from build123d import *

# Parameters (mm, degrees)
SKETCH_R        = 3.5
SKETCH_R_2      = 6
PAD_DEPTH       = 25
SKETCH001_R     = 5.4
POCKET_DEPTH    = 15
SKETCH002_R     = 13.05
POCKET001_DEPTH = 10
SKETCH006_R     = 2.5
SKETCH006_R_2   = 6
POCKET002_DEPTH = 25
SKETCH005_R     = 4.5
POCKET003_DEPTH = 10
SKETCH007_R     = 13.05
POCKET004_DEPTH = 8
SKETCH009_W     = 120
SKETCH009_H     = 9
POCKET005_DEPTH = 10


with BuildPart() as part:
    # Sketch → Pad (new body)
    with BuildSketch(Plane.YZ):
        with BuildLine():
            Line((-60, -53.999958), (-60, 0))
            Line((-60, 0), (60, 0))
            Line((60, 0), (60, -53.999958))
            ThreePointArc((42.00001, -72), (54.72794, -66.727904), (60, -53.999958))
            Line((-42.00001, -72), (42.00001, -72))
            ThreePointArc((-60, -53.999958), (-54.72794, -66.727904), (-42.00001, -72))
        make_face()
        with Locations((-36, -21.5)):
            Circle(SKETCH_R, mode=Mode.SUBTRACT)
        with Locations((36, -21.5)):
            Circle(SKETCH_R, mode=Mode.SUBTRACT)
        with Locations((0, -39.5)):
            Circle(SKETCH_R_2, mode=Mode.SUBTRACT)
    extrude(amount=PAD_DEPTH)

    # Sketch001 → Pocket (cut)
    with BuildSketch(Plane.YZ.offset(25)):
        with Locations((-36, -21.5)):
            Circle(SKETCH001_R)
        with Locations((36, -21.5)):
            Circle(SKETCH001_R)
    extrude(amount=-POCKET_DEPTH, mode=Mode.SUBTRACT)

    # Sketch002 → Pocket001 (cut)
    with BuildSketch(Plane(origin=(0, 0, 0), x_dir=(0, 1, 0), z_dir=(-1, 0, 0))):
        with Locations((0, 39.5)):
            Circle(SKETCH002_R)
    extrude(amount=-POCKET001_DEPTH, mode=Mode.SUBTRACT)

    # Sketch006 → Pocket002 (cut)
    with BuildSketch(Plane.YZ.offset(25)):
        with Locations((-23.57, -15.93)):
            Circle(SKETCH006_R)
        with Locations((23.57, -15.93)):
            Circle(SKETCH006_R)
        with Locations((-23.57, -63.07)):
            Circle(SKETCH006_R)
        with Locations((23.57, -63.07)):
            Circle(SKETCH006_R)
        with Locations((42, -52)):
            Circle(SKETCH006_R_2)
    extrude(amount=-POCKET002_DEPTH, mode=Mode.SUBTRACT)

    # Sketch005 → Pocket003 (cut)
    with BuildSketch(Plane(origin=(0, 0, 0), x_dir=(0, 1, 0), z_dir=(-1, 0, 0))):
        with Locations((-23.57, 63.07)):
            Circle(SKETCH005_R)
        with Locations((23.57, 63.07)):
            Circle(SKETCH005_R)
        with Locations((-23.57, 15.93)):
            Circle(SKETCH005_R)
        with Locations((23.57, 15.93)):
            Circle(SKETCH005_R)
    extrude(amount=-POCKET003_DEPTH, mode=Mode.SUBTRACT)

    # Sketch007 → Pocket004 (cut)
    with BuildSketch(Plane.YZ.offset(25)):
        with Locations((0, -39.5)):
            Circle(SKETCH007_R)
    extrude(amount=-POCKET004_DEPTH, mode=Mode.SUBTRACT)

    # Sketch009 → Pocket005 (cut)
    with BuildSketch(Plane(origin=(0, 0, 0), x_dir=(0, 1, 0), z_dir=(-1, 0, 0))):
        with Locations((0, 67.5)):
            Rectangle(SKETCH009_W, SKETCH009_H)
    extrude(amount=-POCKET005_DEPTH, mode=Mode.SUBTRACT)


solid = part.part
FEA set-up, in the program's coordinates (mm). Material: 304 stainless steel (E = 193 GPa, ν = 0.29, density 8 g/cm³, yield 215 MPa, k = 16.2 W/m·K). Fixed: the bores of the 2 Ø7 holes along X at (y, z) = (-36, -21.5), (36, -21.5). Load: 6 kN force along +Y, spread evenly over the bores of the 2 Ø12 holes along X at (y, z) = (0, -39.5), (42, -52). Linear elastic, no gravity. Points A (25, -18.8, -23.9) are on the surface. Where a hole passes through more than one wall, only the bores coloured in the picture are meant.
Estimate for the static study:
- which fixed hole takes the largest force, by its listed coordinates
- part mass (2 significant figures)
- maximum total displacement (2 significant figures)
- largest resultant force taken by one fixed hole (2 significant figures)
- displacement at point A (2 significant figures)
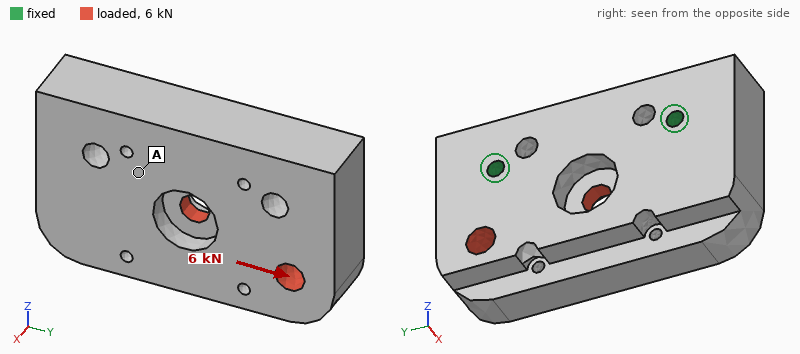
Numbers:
(36, -21.5)
1.5 kg
4.7 µm
4.1 kN
0.95 µm
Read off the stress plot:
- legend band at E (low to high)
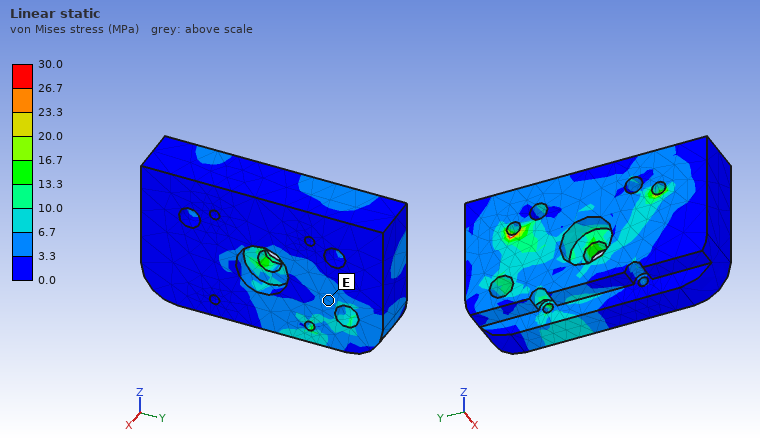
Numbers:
3.3 to 6.7 MPa
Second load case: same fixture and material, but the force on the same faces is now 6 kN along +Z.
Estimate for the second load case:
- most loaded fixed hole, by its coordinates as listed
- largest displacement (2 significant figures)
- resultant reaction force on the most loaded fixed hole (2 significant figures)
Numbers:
(36, -21.5)
13 µm
5.6 kN
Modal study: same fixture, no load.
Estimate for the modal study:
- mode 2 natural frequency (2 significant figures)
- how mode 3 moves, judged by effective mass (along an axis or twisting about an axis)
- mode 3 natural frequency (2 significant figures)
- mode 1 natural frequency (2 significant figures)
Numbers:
5600 Hz
along Y
7700 Hz
2500 Hz
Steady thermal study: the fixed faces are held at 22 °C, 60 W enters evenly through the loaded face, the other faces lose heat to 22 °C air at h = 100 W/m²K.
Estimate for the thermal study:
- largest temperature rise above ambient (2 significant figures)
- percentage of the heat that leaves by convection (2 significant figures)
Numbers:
67 K
73 %
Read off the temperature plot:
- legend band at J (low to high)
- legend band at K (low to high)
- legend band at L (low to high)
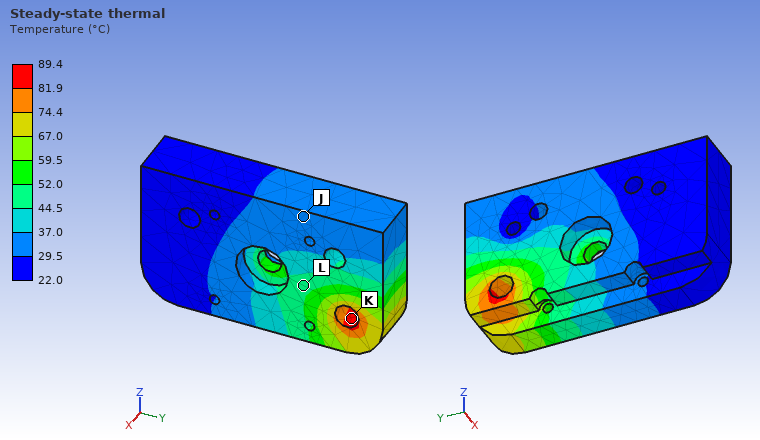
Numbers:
29.5 to 37.0 °C
81.9 to 89.4 °C
44.5 to 52.0 °C
